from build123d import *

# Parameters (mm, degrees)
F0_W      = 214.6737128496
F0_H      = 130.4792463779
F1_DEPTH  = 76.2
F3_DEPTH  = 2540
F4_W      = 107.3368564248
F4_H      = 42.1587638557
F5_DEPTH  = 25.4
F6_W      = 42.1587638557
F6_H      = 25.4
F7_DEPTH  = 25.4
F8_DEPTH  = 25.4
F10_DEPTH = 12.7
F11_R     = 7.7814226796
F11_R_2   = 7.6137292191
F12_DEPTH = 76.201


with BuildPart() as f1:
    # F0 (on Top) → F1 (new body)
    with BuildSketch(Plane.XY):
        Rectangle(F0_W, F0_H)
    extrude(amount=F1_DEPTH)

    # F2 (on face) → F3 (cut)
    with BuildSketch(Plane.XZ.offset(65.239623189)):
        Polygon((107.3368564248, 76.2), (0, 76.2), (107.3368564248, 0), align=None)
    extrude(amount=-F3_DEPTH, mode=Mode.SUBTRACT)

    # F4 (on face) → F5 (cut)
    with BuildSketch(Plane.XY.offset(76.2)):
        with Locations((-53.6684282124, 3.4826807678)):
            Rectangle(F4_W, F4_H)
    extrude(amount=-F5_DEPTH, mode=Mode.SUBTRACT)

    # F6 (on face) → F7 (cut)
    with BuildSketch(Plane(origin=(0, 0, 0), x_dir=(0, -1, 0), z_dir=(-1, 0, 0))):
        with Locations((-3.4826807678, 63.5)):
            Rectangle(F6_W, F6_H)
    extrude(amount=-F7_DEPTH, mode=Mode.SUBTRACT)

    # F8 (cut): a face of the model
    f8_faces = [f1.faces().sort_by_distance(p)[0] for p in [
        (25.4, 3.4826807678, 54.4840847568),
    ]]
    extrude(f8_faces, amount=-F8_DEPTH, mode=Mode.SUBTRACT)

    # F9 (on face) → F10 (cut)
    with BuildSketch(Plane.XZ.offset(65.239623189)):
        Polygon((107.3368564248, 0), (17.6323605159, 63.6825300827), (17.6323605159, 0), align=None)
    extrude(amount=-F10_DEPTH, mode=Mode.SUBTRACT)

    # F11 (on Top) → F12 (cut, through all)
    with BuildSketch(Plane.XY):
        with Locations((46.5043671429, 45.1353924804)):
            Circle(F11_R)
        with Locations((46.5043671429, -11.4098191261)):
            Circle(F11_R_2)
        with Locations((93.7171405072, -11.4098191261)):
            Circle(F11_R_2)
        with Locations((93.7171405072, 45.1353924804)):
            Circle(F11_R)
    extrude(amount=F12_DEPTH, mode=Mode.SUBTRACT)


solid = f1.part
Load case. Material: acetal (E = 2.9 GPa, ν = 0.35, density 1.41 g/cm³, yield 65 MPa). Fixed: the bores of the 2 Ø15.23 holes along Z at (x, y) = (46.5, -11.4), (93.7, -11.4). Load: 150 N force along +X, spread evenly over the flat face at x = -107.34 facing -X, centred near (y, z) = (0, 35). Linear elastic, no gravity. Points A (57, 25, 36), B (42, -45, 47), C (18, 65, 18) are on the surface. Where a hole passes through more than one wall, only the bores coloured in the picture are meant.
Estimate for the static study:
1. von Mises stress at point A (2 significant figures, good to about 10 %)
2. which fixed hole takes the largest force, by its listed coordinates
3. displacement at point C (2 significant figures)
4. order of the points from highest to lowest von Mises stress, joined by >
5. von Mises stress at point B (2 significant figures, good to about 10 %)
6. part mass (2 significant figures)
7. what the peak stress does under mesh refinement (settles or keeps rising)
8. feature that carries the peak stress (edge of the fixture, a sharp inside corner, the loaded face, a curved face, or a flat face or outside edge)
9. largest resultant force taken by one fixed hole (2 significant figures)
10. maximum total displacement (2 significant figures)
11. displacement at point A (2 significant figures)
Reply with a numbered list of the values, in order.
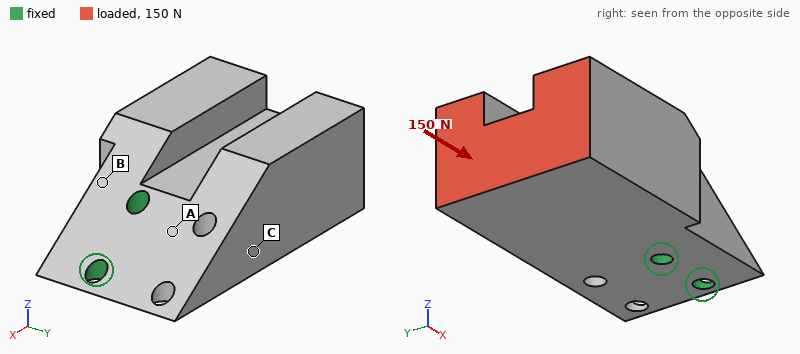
1. 0.052 MPa
2. (46.5, -11.4)
3. 2.7 µm
4. A > B > C
5. 0.032 MPa
6. 2.0 kg
7. keeps rising
8. edge of the fixture
9. 140 N
10. 8.1 µm
11. 1.6 µm
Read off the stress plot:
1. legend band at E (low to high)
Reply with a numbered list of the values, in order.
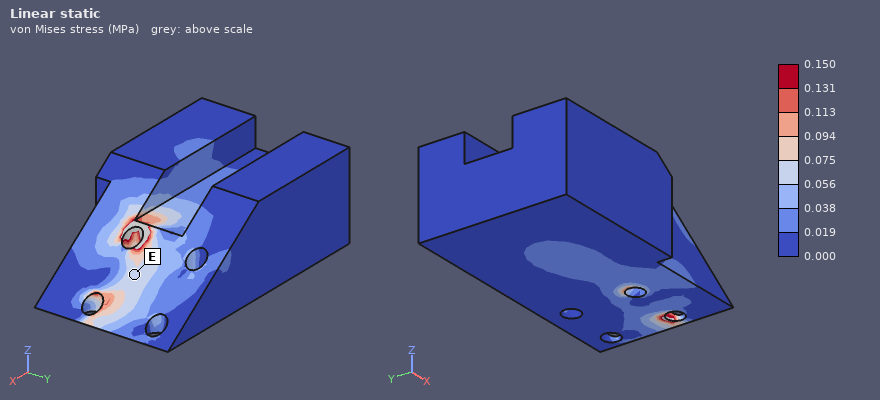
1. 0.056 to 0.075 MPa
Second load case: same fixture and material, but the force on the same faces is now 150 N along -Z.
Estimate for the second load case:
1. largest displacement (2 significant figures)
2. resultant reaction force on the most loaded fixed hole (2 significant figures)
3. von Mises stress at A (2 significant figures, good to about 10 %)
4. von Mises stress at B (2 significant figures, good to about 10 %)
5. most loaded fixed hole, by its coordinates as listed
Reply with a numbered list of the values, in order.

1. 79 µm
2. 210 N
3. 0.33 MPa
4. 0.35 MPa
5. (46.5, -11.4)
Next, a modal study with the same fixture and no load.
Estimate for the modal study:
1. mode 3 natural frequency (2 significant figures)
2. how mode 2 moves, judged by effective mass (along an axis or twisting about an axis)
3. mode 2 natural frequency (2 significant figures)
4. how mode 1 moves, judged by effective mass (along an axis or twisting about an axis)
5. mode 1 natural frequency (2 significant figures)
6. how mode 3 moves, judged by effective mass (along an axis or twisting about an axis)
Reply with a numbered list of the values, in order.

1. 560 Hz
2. along Y
3. 310 Hz
4. along Z
5. 290 Hz
6. twisting about X
